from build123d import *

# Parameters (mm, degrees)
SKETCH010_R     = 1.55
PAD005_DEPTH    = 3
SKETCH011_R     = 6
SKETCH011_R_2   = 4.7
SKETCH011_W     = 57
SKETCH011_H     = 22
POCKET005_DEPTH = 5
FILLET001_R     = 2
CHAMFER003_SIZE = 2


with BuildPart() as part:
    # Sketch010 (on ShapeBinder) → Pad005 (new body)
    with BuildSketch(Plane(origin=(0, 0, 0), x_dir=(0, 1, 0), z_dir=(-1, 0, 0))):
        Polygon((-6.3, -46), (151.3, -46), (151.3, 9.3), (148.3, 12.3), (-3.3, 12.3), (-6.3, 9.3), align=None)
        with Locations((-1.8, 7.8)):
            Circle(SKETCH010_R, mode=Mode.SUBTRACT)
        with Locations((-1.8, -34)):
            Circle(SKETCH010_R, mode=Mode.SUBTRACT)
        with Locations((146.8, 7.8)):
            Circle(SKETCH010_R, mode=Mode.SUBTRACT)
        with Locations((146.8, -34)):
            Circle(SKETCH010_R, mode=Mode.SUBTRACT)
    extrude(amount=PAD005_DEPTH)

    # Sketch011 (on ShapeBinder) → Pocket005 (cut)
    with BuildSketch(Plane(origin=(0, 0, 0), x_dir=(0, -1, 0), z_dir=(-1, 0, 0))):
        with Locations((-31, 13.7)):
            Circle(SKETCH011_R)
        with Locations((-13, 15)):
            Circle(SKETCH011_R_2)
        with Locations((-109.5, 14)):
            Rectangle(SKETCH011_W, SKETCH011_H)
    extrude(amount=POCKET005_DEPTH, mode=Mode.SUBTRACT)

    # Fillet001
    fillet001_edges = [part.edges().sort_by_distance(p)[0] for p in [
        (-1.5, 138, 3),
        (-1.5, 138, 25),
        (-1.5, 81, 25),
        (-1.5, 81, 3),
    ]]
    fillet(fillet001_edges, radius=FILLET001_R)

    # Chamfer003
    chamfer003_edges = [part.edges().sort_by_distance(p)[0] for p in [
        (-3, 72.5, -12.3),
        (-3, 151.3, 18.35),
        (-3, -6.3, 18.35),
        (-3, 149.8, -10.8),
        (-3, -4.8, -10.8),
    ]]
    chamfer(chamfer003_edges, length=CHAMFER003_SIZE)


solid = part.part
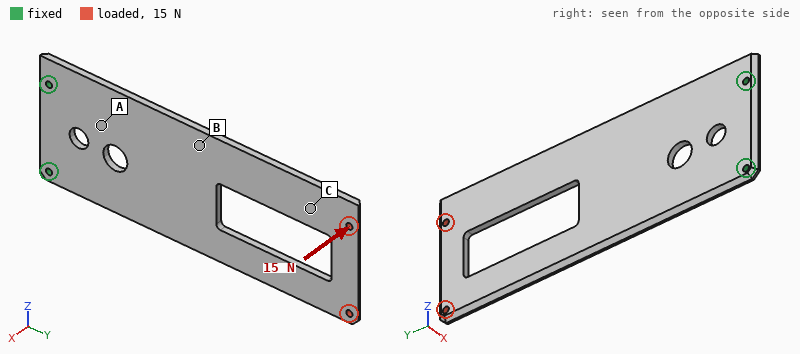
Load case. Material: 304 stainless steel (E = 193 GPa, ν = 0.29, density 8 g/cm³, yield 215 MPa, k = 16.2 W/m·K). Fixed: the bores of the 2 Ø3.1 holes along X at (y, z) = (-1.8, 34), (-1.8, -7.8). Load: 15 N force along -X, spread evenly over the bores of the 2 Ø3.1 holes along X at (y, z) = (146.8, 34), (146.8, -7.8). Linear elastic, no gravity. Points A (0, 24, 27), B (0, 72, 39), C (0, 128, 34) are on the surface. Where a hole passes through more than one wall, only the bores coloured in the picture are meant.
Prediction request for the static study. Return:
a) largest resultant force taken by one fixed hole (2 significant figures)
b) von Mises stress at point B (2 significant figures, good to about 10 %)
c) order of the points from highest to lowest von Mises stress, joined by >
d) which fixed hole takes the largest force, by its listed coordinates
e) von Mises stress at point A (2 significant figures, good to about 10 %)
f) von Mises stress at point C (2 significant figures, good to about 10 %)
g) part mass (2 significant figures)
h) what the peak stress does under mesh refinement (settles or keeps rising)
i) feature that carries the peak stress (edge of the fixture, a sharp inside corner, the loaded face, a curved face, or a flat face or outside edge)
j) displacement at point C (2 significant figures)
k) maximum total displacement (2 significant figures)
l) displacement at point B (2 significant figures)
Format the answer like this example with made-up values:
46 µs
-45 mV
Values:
12 N
15 MPa
A > B > C
(-1.8, 34)
23 MPa
5.7 MPa
180 g
keeps rising
edge of the fixture
0.65 mm
0.86 mm
0.25 mm
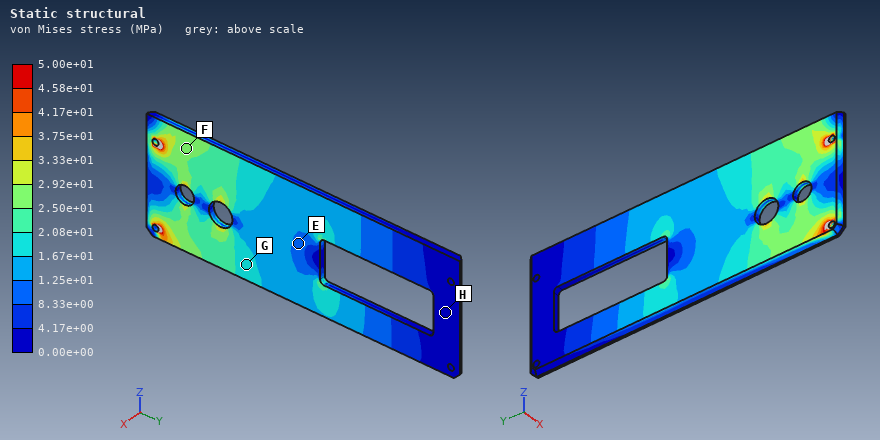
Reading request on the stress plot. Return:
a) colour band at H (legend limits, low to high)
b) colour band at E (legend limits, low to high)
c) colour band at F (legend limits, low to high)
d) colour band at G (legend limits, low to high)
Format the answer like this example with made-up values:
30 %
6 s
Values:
0.00e+00 to 4.17e+00 MPa
8.33e+00 to 1.25e+01 MPa
2.50e+01 to 2.92e+01 MPa
1.67e+01 to 2.08e+01 MPa
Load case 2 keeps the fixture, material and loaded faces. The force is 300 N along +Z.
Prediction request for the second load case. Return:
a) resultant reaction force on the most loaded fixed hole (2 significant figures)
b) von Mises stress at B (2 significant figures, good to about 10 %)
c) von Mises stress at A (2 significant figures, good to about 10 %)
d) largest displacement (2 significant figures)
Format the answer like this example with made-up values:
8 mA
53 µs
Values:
1.1 kN
14 MPa
11 MPa
76 µm
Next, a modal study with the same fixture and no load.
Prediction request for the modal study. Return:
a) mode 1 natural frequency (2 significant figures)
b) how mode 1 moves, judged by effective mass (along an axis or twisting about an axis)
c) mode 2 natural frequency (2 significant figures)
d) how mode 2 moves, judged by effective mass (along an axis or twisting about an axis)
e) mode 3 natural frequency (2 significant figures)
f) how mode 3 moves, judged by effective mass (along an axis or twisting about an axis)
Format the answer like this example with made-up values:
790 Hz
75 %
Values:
110 Hz
along X
530 Hz
twisting about Y
580 Hz
along X
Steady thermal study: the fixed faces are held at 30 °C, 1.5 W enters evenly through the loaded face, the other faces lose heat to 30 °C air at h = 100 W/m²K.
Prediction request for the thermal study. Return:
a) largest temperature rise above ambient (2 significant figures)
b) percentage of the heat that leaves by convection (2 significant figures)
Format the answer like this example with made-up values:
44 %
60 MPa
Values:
15 K
100 %
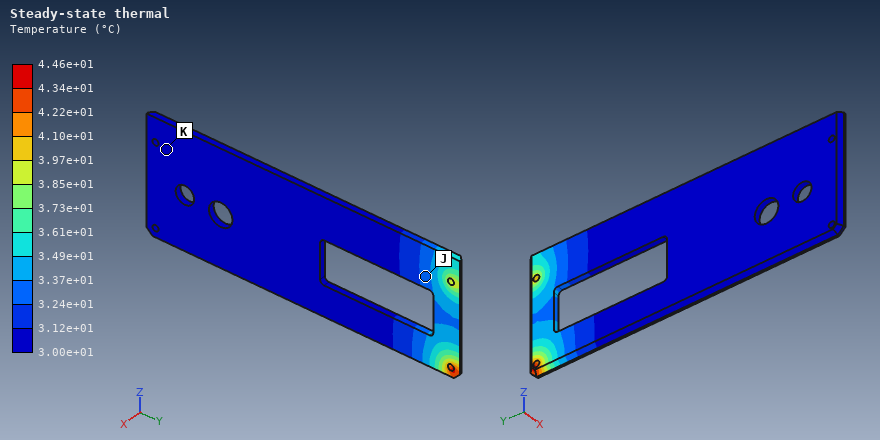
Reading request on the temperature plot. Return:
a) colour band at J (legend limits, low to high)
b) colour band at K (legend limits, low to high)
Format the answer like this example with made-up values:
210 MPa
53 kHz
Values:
3.24e+01 to 3.37e+01 °C
3.00e+01 to 3.12e+01 °C
